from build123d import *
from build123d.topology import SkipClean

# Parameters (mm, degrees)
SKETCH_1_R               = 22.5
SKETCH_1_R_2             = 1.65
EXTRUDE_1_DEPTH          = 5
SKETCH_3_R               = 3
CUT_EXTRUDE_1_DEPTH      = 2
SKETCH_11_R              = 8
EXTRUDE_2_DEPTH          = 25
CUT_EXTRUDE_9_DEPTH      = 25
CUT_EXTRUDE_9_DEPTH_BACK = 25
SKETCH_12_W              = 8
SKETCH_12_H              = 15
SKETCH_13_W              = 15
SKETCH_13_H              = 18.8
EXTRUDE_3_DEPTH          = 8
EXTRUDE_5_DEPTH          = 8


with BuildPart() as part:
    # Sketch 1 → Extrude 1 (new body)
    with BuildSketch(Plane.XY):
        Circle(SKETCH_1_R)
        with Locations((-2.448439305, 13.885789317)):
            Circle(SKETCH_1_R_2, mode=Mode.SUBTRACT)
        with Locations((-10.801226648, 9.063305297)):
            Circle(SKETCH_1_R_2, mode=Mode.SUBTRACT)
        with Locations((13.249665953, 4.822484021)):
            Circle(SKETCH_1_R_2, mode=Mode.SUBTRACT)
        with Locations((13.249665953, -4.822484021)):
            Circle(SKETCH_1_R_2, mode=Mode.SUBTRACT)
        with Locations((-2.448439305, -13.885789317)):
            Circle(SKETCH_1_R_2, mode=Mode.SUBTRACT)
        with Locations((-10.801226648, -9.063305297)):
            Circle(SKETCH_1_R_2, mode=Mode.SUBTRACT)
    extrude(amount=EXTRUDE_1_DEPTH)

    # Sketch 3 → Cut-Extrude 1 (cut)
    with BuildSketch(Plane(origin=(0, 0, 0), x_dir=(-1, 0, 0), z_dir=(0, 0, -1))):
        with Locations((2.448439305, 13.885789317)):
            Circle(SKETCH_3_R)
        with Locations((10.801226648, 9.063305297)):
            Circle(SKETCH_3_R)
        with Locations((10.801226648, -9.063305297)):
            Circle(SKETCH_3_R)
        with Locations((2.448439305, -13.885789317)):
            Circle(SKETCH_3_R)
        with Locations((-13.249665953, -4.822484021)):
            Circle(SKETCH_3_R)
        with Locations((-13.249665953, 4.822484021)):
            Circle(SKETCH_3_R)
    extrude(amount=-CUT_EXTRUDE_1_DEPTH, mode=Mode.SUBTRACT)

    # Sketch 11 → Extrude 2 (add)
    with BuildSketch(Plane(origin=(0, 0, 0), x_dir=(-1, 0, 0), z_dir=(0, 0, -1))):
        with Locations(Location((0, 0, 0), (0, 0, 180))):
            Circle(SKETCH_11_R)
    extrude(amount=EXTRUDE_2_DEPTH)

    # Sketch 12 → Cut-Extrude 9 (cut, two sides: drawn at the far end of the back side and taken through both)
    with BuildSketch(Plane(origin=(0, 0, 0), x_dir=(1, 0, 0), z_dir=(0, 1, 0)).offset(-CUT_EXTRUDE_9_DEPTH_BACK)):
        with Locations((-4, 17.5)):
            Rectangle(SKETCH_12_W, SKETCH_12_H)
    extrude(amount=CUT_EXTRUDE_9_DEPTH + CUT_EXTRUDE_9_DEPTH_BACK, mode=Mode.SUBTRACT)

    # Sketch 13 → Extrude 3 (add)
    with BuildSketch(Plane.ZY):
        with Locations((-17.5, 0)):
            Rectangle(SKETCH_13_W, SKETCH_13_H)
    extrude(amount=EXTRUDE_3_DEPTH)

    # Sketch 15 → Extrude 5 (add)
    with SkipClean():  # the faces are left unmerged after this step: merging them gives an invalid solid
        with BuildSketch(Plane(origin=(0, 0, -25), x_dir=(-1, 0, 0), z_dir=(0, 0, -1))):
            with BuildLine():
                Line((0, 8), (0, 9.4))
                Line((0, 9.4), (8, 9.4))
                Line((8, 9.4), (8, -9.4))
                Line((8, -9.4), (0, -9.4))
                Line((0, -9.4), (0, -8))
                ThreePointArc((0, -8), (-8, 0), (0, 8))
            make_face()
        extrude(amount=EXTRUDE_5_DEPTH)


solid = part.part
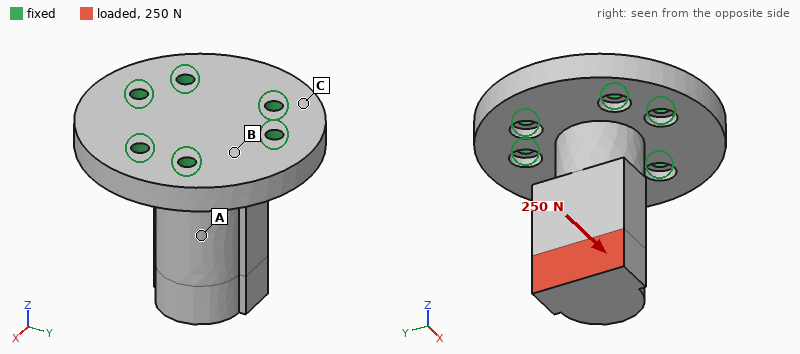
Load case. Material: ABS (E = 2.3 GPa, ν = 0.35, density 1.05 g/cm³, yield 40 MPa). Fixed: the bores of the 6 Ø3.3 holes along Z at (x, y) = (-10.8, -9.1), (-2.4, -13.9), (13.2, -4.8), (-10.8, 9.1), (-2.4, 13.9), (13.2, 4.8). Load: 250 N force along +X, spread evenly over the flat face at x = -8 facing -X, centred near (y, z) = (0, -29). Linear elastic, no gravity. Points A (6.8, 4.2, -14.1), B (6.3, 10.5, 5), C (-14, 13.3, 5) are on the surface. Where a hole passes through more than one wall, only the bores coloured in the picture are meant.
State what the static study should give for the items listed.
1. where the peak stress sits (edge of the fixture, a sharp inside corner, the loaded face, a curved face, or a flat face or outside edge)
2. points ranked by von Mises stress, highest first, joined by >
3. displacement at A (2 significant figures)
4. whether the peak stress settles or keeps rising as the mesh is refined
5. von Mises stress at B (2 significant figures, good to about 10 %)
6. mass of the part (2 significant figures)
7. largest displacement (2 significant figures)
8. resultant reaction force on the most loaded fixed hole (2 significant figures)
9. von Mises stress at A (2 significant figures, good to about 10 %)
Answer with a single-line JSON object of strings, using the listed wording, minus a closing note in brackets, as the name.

{"where the peak stress sits": "edge of the fixture", "points ranked by von Mises stress, highest first, joined by >": "A > B > C", "displacement at A": "0.27 mm", "whether the peak stress settles or keeps rising as the mesh is refined": "keeps rising", "von Mises stress at B": "4.5 MPa", "mass of the part": "16 g", "largest displacement": "0.68 mm", "resultant reaction force on the most loaded fixed hole": "210 N", "von Mises stress at A": "7.1 MPa"}
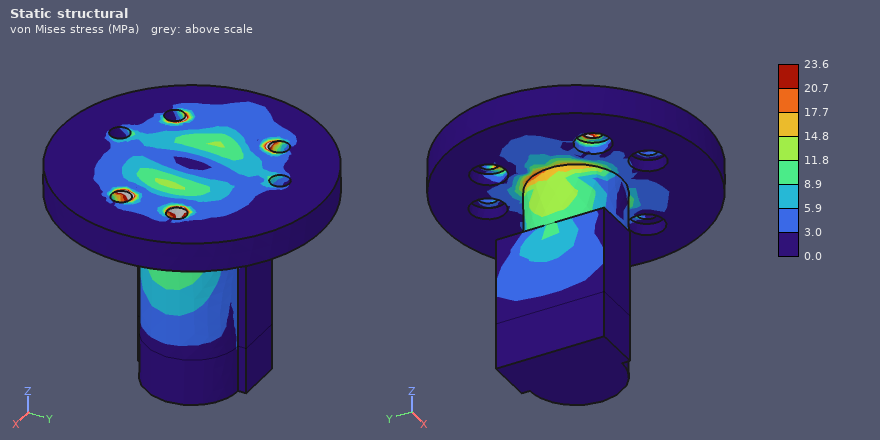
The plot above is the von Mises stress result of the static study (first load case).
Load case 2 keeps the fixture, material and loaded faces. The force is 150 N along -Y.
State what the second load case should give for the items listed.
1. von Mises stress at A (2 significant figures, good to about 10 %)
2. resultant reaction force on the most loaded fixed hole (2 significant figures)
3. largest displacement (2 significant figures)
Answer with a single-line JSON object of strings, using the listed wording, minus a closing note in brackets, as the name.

{"von Mises stress at A": "2.3 MPa", "resultant reaction force on the most loaded fixed hole": "140 N", "largest displacement": "0.45 mm"}
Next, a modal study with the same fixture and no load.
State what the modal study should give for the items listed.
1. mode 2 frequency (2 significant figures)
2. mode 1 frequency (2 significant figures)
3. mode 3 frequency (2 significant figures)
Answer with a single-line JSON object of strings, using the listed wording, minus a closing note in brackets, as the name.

{"mode 2 frequency": "1700 Hz", "mode 1 frequency": "1700 Hz", "mode 3 frequency": "5200 Hz"}
